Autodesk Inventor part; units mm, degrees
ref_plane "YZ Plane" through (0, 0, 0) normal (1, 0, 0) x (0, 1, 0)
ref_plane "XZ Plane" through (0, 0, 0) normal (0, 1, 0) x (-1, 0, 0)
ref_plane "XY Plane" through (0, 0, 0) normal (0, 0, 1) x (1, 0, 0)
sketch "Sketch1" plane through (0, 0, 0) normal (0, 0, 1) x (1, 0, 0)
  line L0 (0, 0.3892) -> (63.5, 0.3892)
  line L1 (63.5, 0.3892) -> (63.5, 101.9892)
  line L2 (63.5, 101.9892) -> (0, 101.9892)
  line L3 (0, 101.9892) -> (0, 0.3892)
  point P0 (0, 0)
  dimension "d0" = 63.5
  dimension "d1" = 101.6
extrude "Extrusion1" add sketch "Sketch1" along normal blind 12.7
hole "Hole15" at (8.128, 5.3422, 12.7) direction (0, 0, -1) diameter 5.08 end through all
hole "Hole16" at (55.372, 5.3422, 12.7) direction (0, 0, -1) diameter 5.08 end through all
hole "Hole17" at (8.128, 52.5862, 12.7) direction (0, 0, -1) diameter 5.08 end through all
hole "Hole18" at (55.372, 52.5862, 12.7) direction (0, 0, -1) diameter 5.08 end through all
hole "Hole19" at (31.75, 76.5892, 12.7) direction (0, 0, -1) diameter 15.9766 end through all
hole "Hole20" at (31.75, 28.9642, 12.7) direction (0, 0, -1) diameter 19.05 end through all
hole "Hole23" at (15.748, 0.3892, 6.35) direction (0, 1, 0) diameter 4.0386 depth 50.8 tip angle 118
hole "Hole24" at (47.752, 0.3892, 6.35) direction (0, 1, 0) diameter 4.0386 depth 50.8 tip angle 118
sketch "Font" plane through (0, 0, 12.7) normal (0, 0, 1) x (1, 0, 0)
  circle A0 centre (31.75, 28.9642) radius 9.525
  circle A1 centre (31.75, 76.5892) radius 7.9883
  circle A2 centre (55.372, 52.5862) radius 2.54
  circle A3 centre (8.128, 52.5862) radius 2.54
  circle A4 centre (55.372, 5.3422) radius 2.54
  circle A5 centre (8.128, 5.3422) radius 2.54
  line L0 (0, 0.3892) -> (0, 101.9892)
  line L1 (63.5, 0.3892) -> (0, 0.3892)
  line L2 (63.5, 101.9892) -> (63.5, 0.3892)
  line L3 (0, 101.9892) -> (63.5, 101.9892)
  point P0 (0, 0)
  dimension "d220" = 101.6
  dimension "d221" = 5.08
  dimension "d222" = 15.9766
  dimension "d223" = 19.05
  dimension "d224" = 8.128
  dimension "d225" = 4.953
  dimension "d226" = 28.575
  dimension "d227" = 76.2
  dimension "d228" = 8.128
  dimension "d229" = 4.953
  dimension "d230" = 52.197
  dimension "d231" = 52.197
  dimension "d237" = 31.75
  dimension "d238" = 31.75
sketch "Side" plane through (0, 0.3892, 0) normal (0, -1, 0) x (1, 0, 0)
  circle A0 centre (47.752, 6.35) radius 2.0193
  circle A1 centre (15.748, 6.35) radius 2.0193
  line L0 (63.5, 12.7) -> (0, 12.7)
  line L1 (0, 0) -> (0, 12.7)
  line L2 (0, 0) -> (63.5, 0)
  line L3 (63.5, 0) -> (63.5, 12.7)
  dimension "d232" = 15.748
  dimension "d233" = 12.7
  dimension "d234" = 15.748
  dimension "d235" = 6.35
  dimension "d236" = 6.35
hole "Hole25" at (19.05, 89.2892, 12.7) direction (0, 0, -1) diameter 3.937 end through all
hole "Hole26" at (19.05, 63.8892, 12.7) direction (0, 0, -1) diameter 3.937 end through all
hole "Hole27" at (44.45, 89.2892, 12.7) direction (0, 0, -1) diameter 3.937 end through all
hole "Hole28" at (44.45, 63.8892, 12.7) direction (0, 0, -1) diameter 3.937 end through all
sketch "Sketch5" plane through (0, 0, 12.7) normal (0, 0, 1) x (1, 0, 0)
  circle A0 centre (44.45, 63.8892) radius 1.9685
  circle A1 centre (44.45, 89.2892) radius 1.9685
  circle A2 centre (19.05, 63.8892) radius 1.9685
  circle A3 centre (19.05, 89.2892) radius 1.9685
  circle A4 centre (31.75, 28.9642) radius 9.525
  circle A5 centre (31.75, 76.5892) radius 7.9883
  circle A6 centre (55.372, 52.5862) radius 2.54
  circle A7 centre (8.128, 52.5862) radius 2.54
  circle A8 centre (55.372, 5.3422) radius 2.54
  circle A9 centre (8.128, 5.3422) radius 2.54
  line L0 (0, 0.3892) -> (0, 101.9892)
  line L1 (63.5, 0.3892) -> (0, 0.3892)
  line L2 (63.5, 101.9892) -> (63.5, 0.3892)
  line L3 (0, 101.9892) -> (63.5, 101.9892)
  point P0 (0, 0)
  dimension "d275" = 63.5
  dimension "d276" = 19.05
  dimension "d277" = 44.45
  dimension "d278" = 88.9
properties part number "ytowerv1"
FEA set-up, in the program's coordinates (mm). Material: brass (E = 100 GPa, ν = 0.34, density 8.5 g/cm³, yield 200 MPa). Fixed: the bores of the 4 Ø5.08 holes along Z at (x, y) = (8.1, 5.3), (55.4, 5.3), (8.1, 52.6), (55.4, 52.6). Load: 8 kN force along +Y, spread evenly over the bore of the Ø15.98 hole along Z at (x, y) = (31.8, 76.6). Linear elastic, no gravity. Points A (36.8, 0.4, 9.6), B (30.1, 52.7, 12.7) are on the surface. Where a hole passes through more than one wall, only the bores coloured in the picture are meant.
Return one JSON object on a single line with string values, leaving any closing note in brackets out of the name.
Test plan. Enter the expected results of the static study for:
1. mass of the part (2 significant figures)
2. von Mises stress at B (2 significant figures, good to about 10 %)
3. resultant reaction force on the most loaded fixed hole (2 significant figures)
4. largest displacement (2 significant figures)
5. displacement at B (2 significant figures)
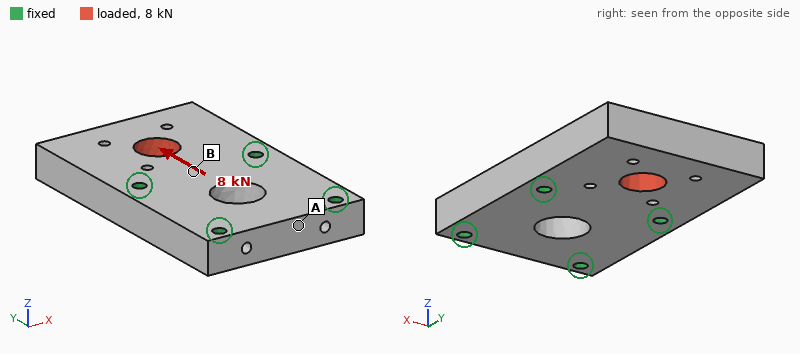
{"mass of the part": "620 g", "von Mises stress at B": "6.1 MPa", "resultant reaction force on the most loaded fixed hole": "3.6 kN", "largest displacement": "7.1 µm", "displacement at B": "2.9 µm"}
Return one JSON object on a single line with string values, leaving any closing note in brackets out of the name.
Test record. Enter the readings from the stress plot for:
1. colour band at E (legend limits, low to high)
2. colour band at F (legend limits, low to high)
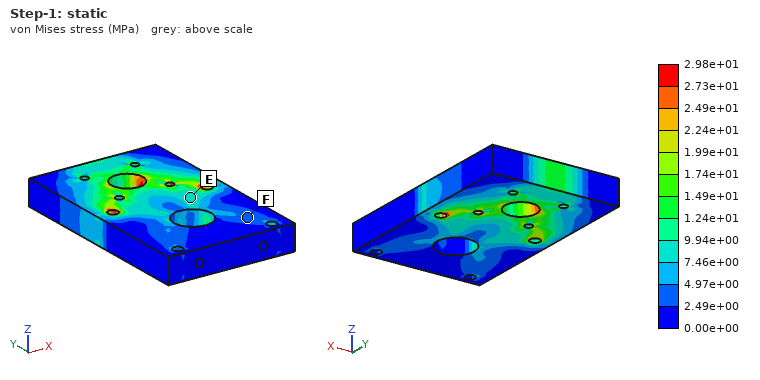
{"colour band at E": "7.46e+00 to 9.94e+00 MPa", "colour band at F": "2.49e+00 to 4.97e+00 MPa"}
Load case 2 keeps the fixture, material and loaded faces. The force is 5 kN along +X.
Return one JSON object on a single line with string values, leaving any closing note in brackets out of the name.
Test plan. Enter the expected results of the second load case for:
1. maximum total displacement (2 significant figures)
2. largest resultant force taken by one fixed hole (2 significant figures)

{"maximum total displacement": "11 µm", "largest resultant force taken by one fixed hole": "3.3 kN"}
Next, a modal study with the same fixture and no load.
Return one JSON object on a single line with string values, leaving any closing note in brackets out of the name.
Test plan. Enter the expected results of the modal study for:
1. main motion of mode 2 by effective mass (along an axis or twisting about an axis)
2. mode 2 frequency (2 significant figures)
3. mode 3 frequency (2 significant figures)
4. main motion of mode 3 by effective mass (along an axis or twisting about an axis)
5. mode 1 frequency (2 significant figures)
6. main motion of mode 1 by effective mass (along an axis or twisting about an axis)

{"main motion of mode 2 by effective mass": "twisting about Y", "mode 2 frequency": "4700 Hz", "mode 3 frequency": "6800 Hz", "main motion of mode 3 by effective mass": "along X", "mode 1 frequency": "2400 Hz", "main motion of mode 1 by effective mass": "along Z"}
